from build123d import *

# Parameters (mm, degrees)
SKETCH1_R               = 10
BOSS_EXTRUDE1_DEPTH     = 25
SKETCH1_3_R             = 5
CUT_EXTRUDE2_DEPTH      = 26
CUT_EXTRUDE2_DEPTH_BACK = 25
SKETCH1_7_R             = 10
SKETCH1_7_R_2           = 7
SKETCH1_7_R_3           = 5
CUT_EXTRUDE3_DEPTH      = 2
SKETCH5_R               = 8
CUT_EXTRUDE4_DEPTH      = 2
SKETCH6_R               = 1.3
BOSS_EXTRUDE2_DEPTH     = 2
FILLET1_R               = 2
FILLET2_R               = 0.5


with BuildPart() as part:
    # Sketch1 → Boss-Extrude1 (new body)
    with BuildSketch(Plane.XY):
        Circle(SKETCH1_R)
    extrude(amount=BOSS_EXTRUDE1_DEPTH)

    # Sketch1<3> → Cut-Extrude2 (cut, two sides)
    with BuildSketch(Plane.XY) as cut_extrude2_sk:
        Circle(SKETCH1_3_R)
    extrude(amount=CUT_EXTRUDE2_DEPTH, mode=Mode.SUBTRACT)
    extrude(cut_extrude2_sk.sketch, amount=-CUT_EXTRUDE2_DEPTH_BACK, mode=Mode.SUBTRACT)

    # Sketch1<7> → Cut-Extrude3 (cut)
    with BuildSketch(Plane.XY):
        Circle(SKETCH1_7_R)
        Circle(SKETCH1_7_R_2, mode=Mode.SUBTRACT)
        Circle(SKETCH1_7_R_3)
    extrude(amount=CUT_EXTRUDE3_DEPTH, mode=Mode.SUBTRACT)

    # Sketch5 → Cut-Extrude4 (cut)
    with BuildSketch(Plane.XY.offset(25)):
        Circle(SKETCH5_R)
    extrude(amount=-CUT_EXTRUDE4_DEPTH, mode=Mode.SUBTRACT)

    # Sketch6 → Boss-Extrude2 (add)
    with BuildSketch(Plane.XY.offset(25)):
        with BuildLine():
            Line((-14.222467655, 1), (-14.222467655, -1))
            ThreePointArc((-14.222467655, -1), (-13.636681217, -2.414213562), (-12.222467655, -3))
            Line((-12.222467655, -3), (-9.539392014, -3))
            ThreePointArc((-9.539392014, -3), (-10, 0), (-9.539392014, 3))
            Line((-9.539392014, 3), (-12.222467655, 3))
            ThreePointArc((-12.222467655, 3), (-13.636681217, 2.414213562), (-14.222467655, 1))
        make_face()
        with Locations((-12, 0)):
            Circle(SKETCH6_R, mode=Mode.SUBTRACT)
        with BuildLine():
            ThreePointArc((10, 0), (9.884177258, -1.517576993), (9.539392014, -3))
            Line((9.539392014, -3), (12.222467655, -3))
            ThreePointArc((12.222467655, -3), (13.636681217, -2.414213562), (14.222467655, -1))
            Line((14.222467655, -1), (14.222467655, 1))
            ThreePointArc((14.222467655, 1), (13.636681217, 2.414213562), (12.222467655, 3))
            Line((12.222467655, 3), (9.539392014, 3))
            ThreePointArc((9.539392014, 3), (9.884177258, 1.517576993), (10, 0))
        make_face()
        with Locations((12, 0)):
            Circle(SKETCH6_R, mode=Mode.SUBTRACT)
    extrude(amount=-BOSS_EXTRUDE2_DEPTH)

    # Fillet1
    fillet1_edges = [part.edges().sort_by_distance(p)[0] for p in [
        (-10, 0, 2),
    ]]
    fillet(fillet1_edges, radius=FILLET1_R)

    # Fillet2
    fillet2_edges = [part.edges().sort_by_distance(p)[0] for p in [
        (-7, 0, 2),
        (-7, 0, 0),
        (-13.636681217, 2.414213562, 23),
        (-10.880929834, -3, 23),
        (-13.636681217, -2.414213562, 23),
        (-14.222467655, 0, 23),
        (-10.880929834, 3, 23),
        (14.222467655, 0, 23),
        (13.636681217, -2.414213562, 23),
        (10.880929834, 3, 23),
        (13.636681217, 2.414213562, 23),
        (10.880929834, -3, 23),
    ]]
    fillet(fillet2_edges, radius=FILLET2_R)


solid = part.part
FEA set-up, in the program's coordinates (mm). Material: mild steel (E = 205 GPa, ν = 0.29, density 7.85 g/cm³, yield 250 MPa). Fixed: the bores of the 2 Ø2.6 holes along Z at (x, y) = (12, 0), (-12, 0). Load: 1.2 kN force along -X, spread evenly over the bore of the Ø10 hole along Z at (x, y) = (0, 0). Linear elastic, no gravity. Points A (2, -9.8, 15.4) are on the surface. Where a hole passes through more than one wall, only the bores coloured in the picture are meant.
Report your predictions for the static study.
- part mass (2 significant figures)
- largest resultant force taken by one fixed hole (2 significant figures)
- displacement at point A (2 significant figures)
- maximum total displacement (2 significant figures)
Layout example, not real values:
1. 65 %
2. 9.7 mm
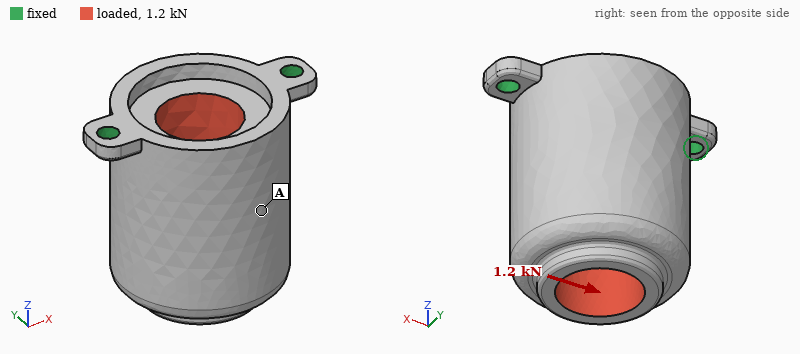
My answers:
1. 42 g
2. 940 N
3. 3.9 µm
4. 10 µm
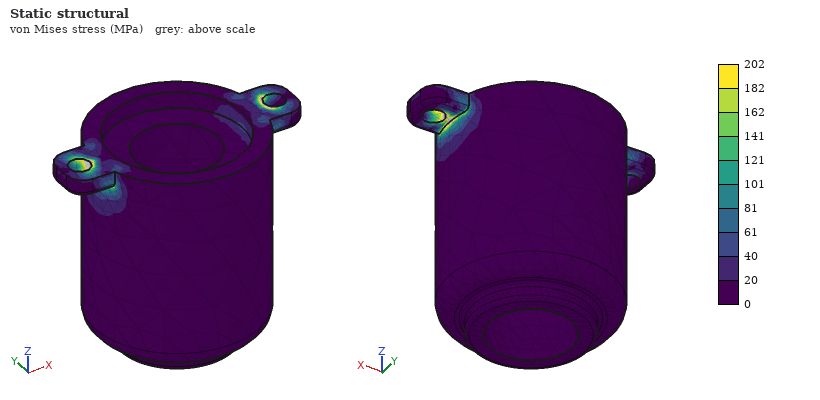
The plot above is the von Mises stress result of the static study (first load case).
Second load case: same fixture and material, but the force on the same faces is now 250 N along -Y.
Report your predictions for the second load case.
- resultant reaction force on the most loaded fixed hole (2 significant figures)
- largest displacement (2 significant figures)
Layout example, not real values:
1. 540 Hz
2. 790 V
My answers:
1. 130 N
2. 61 µm
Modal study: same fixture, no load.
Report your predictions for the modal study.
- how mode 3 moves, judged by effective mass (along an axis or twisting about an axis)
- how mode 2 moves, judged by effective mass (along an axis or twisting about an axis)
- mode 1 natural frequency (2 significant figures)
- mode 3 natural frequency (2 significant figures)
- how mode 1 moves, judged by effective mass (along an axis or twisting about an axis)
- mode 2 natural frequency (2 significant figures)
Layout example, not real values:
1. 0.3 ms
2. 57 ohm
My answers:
1. along Z
2. along X
3. 2000 Hz
4. 15 kHz
5. along Y
6. 11 kHz
